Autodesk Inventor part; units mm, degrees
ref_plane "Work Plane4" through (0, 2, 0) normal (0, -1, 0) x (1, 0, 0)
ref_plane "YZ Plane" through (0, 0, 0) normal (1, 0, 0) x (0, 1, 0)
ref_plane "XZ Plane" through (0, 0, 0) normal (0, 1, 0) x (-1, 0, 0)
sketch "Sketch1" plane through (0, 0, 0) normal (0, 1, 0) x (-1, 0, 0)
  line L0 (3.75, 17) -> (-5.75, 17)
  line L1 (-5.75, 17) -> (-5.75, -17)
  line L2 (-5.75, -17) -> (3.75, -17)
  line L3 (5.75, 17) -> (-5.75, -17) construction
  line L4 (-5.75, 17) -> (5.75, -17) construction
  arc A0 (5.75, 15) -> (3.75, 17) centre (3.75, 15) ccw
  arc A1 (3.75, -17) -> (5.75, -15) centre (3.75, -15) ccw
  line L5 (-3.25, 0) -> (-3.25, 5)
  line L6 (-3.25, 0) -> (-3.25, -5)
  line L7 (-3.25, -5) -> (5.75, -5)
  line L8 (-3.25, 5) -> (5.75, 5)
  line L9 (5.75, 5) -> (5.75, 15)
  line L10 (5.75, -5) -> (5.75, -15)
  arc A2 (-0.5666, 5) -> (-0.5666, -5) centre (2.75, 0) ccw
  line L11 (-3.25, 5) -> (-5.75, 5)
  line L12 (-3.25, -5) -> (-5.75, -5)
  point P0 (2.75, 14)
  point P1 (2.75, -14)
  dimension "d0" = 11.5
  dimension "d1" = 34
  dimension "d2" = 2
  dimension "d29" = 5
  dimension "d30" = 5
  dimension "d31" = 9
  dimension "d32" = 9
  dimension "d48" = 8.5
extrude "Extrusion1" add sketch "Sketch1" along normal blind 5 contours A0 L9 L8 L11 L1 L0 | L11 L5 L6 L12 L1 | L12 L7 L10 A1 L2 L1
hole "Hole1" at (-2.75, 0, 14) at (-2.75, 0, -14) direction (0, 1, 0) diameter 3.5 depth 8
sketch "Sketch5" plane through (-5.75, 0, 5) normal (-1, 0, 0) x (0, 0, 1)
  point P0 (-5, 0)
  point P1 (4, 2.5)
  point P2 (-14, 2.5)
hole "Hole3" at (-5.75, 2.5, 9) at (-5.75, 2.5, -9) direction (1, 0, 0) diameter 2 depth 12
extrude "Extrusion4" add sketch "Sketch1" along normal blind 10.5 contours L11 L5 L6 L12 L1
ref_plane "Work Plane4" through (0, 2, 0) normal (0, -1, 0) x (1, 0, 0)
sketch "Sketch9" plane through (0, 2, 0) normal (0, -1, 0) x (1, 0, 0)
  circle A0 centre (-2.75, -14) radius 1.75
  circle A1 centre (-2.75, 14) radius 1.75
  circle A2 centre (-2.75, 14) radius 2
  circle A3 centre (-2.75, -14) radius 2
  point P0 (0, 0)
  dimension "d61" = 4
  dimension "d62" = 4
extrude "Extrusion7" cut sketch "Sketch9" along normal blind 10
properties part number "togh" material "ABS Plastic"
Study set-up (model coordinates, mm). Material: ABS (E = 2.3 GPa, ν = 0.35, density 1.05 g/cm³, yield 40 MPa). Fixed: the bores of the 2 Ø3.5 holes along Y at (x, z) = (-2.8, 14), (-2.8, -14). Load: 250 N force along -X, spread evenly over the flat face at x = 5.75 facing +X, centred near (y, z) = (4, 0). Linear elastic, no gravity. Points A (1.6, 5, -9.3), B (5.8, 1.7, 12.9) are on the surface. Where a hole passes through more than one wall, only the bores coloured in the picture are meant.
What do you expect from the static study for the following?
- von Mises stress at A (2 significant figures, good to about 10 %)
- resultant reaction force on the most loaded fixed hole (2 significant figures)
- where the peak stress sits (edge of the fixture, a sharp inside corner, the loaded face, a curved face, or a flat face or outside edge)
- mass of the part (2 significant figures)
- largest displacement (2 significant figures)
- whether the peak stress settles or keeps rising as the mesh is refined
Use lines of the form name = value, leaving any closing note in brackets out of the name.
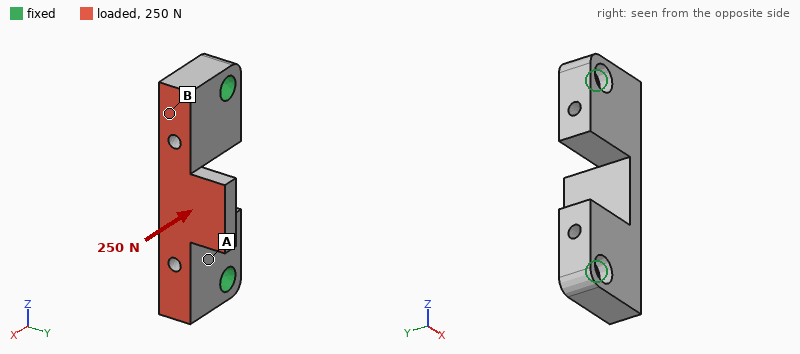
von Mises stress at A = 11 MPa
resultant reaction force on the most loaded fixed hole = 150 N
where the peak stress sits = a sharp inside corner
mass of the part = 1.5 g
largest displacement = 0.40 mm
whether the peak stress settles or keeps rising as the mesh is refined = keeps rising
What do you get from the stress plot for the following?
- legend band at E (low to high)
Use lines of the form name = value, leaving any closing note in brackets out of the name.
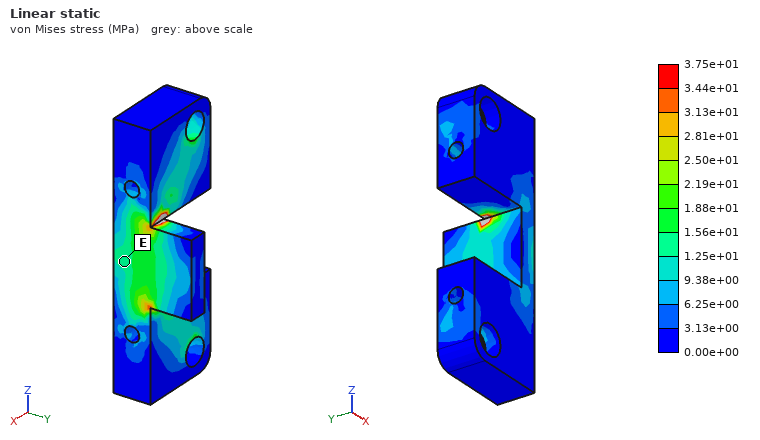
legend band at E = 1.25e+01 to 1.56e+01 MPa
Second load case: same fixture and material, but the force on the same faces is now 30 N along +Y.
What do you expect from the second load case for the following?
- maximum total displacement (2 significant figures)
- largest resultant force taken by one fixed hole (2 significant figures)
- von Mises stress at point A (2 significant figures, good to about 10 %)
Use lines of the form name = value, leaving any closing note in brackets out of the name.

maximum total displacement = 74 µm
largest resultant force taken by one fixed hole = 15 N
von Mises stress at point A = 1.6 MPa
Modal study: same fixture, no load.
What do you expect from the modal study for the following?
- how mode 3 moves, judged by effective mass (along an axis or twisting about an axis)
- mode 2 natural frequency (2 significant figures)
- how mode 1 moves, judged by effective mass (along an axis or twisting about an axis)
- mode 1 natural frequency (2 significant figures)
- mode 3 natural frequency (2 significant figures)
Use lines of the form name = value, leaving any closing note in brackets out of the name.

how mode 3 moves, judged by effective mass = along Z
mode 2 natural frequency = 7100 Hz
how mode 1 moves, judged by effective mass = along Y
mode 1 natural frequency = 5100 Hz
mode 3 natural frequency = 8300 Hz
